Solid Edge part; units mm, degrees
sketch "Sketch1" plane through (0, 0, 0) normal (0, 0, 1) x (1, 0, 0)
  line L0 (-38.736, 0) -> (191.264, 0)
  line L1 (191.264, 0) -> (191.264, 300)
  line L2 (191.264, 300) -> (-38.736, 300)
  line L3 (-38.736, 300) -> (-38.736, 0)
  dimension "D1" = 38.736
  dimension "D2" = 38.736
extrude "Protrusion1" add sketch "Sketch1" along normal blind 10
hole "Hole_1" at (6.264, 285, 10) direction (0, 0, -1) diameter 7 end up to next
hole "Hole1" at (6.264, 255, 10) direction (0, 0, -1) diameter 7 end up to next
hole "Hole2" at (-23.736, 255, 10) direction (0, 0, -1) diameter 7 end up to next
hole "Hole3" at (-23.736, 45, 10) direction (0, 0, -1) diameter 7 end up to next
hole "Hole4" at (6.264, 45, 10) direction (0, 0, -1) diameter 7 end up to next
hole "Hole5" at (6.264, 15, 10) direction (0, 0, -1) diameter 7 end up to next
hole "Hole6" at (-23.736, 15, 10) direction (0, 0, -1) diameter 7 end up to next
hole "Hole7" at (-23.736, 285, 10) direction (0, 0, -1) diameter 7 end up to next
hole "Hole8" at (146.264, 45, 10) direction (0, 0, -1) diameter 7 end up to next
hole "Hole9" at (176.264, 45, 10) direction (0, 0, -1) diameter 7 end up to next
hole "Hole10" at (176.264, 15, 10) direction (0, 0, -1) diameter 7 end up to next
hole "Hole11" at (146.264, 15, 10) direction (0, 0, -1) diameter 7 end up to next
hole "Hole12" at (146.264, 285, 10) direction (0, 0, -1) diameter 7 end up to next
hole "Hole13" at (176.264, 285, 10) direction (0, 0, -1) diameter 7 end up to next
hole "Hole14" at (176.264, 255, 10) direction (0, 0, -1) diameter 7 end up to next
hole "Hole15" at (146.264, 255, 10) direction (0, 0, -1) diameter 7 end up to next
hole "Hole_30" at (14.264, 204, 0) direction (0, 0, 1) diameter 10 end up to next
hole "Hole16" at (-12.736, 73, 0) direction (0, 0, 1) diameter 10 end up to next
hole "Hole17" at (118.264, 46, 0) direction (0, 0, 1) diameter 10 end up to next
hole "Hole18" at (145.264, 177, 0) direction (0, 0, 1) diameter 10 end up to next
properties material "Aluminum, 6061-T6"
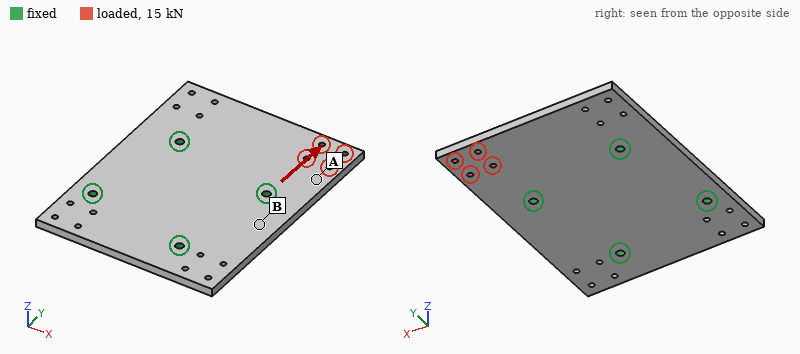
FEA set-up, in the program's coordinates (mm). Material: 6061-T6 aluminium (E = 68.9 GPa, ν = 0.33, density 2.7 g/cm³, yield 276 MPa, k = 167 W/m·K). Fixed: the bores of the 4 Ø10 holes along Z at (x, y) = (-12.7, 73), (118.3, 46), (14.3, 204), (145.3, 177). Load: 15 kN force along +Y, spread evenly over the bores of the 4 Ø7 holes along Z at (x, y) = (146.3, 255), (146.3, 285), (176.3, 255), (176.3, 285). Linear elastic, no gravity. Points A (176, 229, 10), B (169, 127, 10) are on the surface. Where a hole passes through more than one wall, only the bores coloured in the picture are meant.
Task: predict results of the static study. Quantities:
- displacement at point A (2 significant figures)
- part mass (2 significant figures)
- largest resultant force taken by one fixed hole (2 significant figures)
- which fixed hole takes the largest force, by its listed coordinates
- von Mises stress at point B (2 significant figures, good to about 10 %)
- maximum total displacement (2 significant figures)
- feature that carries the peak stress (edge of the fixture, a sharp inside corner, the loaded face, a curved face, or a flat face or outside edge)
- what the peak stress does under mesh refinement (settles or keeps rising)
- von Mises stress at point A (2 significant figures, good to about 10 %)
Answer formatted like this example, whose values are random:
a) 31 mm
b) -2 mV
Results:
a) 28 µm
b) 1.8 kg
c) 12 kN
d) (145.3, 177)
e) 5.7 MPa
f) 50 µm
g) edge of the fixture
h) keeps rising
i) 22 MPa
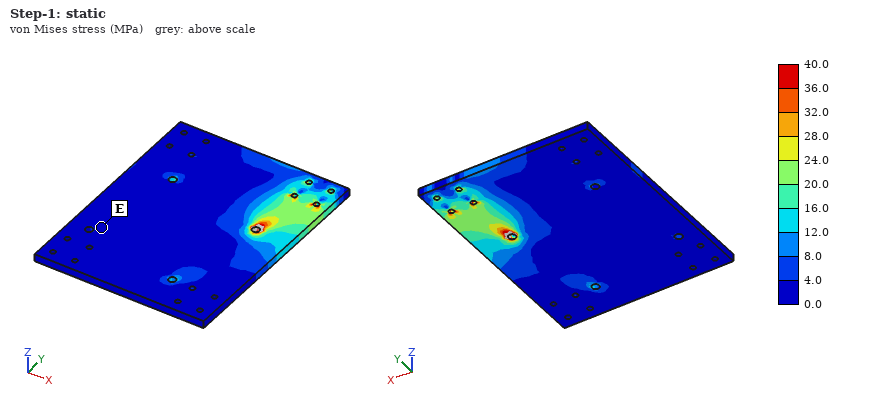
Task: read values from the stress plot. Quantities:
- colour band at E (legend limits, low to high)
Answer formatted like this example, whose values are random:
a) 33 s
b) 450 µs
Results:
a) 0.0 to 4.0 MPa
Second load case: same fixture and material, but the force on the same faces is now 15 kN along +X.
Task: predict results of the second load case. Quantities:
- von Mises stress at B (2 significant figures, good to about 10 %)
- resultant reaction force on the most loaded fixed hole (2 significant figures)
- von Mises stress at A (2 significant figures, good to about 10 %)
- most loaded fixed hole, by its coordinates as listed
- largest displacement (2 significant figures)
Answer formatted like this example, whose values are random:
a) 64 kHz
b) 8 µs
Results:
a) 5.1 MPa
b) 11 kN
c) 9.4 MPa
d) (14.3, 204)
e) 69 µm
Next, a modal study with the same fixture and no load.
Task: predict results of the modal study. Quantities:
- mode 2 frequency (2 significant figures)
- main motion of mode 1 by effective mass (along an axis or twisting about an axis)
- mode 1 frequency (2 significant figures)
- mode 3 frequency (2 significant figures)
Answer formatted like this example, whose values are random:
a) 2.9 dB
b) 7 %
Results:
a) 1000 Hz
b) along Z
c) 600 Hz
d) 1400 Hz
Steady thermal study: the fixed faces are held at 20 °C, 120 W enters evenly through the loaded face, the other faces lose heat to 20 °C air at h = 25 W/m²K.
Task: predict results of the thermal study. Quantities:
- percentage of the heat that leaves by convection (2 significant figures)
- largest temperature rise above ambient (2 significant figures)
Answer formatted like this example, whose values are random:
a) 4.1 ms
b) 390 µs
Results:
a) 26 %
b) 61 K
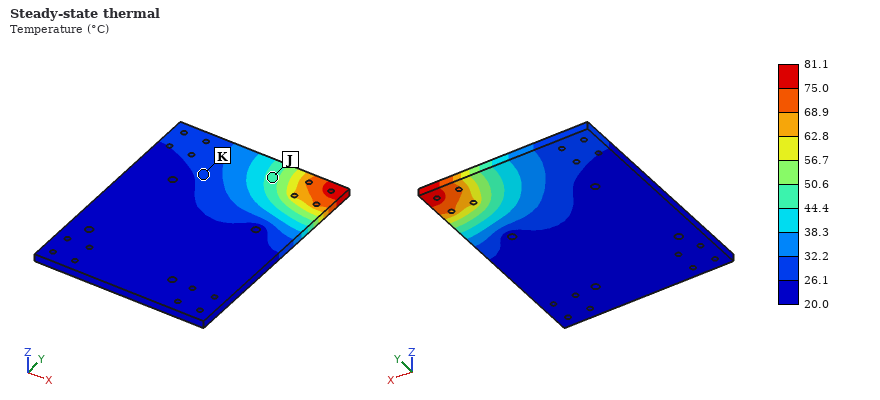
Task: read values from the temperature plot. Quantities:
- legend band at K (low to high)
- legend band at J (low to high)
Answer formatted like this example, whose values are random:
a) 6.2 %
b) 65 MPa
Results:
a) 26.1 to 32.2 °C
b) 44.4 to 50.6 °C
